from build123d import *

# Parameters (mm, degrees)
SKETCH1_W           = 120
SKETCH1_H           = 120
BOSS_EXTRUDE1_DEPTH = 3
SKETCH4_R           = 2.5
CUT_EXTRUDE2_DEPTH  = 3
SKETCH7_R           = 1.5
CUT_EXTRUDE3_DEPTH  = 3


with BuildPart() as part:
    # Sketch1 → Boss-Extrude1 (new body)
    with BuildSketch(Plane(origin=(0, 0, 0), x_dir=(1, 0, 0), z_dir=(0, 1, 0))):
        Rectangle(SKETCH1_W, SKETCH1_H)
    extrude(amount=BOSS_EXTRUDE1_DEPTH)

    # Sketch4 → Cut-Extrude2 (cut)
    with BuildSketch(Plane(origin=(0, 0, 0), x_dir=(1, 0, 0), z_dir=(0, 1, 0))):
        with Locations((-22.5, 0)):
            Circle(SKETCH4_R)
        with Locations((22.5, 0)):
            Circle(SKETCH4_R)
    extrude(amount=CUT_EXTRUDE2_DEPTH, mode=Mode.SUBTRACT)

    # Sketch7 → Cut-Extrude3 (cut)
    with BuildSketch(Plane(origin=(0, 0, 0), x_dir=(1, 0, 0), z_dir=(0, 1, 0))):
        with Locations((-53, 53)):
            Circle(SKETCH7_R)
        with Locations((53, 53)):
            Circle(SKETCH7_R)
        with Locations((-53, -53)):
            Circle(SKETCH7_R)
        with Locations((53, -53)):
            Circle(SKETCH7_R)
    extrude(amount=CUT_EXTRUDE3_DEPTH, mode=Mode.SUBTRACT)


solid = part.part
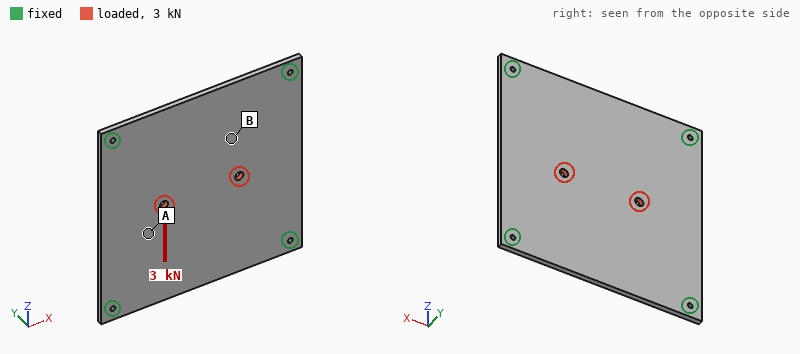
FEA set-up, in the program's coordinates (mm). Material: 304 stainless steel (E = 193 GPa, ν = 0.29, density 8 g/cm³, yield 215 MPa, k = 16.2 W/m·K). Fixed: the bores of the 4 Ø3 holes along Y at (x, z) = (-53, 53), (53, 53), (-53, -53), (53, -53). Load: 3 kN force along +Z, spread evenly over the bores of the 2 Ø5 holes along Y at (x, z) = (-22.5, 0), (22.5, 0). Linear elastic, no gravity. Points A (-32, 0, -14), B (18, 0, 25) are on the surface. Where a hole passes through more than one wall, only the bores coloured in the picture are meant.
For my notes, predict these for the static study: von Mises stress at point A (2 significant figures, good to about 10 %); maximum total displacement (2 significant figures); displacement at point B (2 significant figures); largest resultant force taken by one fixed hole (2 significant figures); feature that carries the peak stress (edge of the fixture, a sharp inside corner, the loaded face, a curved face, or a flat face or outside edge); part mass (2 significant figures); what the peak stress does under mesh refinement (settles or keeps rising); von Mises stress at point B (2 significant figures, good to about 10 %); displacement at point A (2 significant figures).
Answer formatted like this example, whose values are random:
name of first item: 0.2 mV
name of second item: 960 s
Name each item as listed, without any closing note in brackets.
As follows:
von Mises stress at point A: 11 MPa
maximum total displacement: 4.8 µm
displacement at point B: 3.4 µm
largest resultant force taken by one fixed hole: 820 N
feature that carries the peak stress: edge of the fixture
part mass: 340 g
what the peak stress does under mesh refinement: keeps rising
von Mises stress at point B: 4.7 MPa
displacement at point A: 3.0 µm
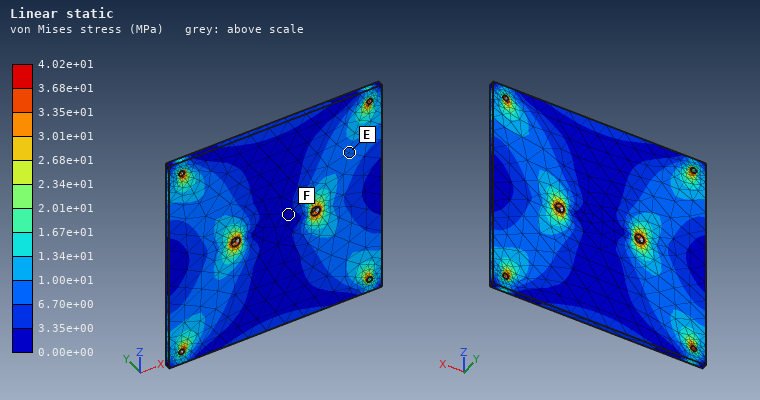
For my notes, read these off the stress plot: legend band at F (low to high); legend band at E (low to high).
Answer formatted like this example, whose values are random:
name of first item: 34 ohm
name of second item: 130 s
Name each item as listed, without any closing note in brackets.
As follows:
legend band at F: 0.00e+00 to 3.35e+00 MPa
legend band at E: 6.70e+00 to 1.00e+01 MPa
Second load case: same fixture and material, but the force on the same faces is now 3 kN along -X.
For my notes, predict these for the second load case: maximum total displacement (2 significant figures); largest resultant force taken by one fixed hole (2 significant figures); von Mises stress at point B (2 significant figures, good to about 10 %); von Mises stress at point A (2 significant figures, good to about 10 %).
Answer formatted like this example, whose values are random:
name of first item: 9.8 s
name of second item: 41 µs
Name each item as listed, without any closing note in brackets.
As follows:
maximum total displacement: 5.7 µm
largest resultant force taken by one fixed hole: 850 N
von Mises stress at point B: 8.4 MPa
von Mises stress at point A: 8.8 MPa
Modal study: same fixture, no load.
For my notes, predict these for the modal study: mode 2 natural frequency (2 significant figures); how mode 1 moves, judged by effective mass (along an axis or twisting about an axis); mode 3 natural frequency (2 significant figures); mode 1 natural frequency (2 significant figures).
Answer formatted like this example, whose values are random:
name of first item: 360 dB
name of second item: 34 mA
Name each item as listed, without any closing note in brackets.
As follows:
mode 2 natural frequency: 1400 Hz
how mode 1 moves, judged by effective mass: along Y
mode 3 natural frequency: 1400 Hz
mode 1 natural frequency: 800 Hz
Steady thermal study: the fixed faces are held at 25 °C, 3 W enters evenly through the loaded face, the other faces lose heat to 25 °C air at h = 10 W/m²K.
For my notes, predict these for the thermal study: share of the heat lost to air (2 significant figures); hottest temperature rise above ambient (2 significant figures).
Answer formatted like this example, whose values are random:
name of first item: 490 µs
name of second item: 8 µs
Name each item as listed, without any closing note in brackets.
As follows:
share of the heat lost to air: 65 %
hottest temperature rise above ambient: 19 K
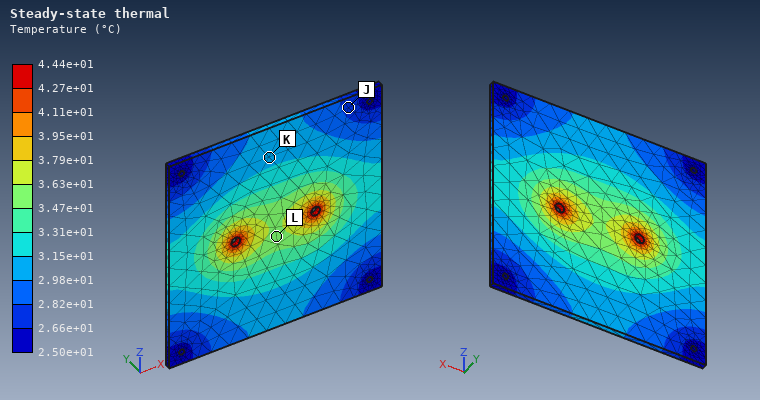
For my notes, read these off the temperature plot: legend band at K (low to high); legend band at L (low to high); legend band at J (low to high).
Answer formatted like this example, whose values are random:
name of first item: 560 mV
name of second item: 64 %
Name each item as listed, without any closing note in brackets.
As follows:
legend band at K: 2.98e+01 to 3.15e+01 °C
legend band at L: 3.47e+01 to 3.63e+01 °C
legend band at J: 2.66e+01 to 2.82e+01 °C
